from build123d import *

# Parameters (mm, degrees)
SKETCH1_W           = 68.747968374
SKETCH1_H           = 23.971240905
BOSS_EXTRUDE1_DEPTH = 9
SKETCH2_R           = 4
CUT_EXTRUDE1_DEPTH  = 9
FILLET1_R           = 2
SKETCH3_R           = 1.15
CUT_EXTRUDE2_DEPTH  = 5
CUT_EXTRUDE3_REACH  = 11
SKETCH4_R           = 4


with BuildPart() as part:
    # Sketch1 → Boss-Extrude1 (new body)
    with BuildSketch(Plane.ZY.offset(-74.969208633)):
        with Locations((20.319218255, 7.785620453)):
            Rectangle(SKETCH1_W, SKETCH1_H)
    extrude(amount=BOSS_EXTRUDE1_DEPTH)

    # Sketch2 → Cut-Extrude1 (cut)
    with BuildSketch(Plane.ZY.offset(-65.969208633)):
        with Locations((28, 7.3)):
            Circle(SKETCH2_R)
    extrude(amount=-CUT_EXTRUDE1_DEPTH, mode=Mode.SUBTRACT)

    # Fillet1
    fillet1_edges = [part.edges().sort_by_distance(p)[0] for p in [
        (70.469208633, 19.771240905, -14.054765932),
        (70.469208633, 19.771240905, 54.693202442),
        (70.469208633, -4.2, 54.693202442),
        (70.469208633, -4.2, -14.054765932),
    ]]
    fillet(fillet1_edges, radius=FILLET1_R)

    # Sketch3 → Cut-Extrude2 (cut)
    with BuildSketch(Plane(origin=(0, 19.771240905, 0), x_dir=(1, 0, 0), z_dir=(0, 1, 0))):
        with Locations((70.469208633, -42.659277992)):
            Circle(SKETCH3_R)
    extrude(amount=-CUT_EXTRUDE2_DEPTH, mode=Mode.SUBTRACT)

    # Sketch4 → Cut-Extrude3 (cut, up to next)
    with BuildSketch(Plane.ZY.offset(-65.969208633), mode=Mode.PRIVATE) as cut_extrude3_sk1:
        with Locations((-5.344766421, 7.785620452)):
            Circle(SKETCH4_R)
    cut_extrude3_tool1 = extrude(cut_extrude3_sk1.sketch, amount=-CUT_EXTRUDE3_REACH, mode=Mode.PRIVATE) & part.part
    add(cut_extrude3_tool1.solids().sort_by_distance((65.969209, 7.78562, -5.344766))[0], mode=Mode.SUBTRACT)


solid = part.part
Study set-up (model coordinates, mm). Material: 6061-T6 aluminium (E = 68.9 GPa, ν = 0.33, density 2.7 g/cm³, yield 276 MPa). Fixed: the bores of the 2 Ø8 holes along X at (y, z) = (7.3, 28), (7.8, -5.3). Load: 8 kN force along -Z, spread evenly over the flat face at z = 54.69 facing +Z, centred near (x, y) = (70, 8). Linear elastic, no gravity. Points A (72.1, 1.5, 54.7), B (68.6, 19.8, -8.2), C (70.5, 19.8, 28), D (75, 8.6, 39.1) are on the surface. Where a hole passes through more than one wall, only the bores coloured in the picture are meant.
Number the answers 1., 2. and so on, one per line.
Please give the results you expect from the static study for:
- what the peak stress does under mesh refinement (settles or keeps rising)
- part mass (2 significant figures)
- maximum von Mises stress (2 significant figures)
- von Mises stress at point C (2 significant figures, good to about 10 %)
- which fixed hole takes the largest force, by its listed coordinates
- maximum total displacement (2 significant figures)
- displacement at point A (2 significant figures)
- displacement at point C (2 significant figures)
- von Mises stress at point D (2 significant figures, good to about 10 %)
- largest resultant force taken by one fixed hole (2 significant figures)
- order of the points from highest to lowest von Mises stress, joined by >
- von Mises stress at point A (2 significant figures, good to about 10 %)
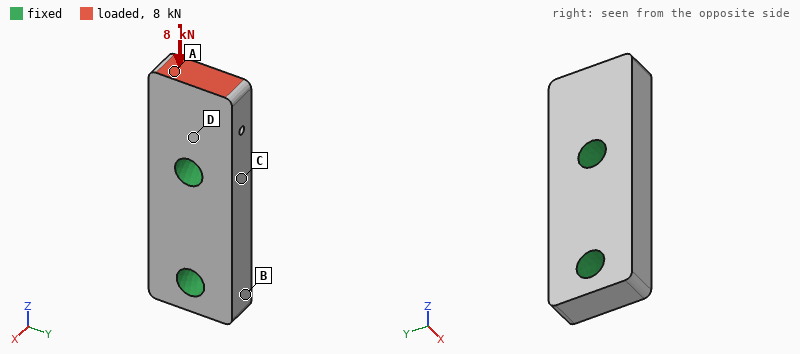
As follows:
1. settles
2. 37 g
3. 89 MPa
4. 22 MPa
5. (7.3, 28)
6. 17 µm
7. 15 µm
8. 4.2 µm
9. 51 MPa
10. 7.4 kN
11. D > A > C > B
12. 38 MPa
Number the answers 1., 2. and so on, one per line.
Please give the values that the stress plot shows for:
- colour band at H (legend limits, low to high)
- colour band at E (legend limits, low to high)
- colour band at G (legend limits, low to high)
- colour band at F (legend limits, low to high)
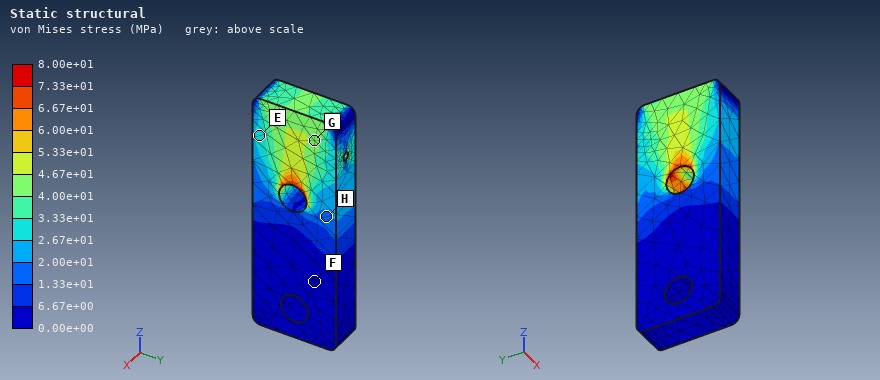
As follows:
1. 1.33e+01 to 2.00e+01 MPa
2. 2.67e+01 to 3.33e+01 MPa
3. 4.00e+01 to 4.67e+01 MPa
4. 0.00e+00 to 6.67e+00 MPa
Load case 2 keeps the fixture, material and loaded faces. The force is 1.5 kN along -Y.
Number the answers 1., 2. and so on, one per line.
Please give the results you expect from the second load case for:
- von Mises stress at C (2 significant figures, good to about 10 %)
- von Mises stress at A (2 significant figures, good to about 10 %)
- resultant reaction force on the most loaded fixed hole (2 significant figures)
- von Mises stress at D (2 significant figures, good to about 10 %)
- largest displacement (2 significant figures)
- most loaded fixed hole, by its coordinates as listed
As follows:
1. 33 MPa
2. 15 MPa
3. 2.0 kN
4. 19 MPa
5. 32 µm
6. (7.3, 28)
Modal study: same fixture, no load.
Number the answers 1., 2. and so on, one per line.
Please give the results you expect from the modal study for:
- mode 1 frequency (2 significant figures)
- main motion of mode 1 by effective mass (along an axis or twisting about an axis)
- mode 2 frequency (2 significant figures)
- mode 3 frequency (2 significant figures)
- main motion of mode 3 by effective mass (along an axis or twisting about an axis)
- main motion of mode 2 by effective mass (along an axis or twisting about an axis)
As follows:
1. 11 kHz
2. along X
3. 16 kHz
4. 20 kHz
5. twisting about Z
6. along Y
